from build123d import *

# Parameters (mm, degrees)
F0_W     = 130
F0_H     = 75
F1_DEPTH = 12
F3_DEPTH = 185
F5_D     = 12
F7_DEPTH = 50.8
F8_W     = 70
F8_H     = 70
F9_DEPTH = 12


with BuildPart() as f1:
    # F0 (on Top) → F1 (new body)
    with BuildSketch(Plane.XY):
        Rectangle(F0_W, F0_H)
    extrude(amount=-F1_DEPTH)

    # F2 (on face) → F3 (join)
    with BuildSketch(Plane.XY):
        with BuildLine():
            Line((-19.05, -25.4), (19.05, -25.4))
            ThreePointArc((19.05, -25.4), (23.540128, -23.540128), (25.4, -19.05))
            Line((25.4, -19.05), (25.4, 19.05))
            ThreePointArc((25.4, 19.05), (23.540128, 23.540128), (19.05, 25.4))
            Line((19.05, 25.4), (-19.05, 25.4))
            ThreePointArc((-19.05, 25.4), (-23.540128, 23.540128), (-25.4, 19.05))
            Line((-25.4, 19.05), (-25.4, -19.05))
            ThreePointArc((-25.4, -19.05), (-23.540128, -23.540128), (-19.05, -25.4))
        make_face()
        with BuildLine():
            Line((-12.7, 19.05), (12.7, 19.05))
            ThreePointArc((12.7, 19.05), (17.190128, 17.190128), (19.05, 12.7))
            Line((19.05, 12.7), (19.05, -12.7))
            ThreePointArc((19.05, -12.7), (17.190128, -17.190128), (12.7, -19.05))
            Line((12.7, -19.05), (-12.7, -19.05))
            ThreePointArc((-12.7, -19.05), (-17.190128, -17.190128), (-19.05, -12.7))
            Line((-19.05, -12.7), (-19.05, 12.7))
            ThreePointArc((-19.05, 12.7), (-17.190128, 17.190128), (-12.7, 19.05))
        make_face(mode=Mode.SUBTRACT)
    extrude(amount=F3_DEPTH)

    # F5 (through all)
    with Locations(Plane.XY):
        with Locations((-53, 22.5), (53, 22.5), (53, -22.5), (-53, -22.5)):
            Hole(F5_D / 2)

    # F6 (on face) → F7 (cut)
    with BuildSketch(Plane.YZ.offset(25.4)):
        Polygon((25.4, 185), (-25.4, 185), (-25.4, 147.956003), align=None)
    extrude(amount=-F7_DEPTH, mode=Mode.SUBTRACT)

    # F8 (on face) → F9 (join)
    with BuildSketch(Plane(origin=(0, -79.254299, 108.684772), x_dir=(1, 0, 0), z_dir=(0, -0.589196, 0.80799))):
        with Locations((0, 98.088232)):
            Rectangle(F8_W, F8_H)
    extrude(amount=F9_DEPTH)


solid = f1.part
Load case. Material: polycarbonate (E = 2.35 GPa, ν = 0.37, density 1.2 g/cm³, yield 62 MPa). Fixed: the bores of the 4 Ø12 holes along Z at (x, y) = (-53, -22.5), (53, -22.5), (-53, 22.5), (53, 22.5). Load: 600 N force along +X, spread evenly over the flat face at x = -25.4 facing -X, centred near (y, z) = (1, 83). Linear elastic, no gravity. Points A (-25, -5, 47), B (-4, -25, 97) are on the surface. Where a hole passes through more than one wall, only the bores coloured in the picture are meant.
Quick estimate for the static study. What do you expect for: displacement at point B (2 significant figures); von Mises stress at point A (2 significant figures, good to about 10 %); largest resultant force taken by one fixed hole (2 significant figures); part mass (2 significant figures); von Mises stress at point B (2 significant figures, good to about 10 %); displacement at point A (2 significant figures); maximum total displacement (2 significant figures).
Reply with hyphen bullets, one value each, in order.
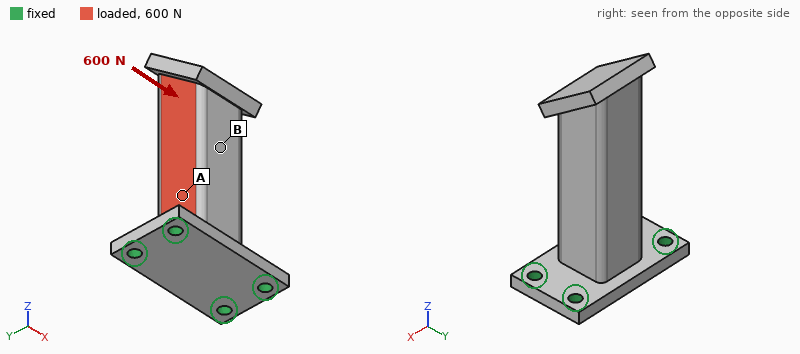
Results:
- 0.57 mm
- 2.2 MPa
- 380 N
- 430 g
- 1.0 MPa
- 0.32 mm
- 1.2 mm
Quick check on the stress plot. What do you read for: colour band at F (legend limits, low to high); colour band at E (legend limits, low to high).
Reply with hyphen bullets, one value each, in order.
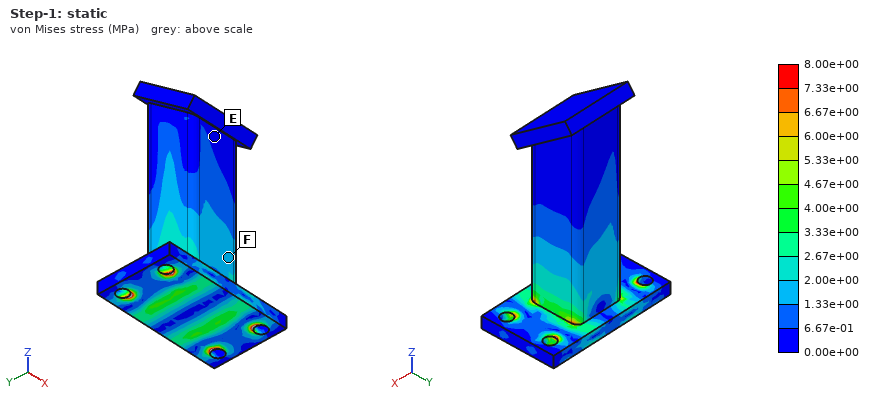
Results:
- 1.33e+00 to 2.00e+00 MPa
- 0.00e+00 to 6.67e-01 MPa
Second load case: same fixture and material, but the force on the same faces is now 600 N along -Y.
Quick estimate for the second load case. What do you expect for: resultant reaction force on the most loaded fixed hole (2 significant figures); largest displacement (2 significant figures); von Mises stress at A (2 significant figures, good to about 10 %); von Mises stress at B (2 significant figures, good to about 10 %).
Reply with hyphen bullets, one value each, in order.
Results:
- 610 N
- 2.4 mm
- 2.4 MPa
- 0.87 MPa
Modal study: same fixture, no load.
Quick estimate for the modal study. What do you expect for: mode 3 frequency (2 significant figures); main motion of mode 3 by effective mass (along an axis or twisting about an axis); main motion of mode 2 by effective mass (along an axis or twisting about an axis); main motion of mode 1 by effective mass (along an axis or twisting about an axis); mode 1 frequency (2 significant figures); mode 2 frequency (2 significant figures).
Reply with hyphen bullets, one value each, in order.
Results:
- 790 Hz
- along Z
- along X
- along Y
- 160 Hz
- 210 Hz
